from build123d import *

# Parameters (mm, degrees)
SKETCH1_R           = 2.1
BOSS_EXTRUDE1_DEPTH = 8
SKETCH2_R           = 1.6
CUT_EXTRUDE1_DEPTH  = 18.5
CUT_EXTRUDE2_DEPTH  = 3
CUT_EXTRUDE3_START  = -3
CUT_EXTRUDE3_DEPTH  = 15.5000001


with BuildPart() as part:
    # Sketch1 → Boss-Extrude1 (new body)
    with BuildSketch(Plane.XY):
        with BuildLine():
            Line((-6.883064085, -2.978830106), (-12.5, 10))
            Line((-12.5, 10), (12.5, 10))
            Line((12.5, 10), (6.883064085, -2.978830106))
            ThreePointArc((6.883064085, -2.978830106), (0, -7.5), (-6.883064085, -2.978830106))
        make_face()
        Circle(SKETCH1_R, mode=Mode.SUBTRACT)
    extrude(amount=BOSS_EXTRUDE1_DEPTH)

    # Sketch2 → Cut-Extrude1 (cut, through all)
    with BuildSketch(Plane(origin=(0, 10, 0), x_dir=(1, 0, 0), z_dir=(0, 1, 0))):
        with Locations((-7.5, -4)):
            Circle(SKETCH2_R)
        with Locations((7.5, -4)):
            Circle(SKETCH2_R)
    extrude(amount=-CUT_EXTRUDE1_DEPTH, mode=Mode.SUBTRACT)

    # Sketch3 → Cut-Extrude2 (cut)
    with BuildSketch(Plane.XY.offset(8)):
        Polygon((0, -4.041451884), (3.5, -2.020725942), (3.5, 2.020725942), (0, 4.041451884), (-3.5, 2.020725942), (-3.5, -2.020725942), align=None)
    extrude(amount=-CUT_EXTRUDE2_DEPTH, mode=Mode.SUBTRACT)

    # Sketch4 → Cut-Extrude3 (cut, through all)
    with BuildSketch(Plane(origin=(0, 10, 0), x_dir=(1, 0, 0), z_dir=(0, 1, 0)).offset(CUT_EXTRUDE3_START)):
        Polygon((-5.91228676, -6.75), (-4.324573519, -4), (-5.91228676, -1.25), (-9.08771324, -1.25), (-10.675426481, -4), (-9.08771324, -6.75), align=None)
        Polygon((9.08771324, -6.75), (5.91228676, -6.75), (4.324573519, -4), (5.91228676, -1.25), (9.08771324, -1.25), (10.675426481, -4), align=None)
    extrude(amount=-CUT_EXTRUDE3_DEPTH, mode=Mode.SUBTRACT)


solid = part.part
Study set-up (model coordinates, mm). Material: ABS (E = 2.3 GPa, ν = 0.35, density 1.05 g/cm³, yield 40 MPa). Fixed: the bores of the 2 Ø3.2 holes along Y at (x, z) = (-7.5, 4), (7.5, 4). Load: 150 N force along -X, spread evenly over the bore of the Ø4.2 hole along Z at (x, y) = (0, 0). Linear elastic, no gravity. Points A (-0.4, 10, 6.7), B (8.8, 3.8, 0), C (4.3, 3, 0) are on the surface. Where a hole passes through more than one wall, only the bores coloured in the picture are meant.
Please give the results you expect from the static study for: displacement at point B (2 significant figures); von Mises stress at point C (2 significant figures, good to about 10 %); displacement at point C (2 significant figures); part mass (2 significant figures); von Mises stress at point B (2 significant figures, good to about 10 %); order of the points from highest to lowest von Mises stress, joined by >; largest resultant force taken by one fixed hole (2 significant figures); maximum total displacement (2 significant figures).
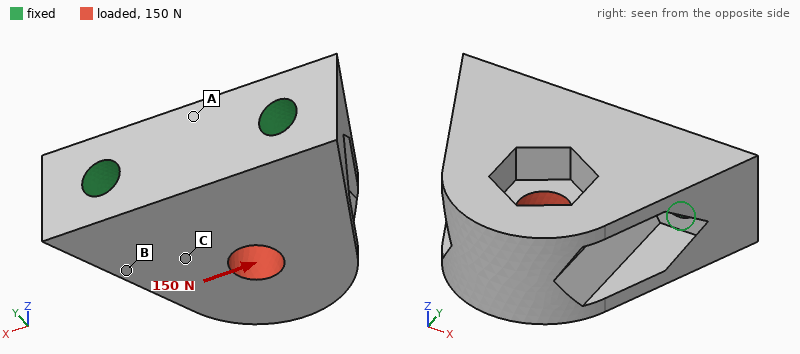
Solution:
22 µm
3.9 MPa
21 µm
1.8 g
2.2 MPa
C > B > A
110 N
54 µm
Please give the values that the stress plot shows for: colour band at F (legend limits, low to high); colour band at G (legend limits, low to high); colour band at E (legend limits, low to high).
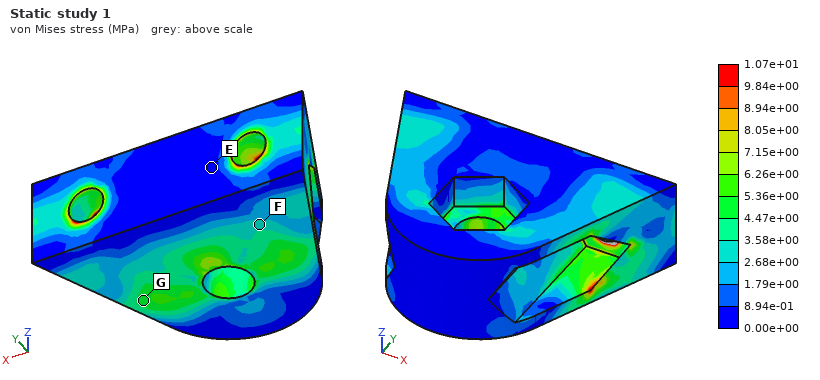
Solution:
2.68e+00 to 3.58e+00 MPa
4.47e+00 to 5.36e+00 MPa
0.00e+00 to 8.94e-01 MPa
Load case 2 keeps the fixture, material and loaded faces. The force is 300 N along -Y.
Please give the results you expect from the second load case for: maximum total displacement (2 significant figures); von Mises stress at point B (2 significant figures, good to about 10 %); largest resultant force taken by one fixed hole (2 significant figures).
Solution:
0.11 mm
5.8 MPa
160 N
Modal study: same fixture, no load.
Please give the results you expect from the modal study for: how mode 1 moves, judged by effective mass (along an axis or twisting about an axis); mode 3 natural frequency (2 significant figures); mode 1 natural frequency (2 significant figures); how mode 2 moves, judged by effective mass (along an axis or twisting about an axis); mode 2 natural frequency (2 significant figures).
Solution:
along Z
11 kHz
4100 Hz
along X
9100 Hz
